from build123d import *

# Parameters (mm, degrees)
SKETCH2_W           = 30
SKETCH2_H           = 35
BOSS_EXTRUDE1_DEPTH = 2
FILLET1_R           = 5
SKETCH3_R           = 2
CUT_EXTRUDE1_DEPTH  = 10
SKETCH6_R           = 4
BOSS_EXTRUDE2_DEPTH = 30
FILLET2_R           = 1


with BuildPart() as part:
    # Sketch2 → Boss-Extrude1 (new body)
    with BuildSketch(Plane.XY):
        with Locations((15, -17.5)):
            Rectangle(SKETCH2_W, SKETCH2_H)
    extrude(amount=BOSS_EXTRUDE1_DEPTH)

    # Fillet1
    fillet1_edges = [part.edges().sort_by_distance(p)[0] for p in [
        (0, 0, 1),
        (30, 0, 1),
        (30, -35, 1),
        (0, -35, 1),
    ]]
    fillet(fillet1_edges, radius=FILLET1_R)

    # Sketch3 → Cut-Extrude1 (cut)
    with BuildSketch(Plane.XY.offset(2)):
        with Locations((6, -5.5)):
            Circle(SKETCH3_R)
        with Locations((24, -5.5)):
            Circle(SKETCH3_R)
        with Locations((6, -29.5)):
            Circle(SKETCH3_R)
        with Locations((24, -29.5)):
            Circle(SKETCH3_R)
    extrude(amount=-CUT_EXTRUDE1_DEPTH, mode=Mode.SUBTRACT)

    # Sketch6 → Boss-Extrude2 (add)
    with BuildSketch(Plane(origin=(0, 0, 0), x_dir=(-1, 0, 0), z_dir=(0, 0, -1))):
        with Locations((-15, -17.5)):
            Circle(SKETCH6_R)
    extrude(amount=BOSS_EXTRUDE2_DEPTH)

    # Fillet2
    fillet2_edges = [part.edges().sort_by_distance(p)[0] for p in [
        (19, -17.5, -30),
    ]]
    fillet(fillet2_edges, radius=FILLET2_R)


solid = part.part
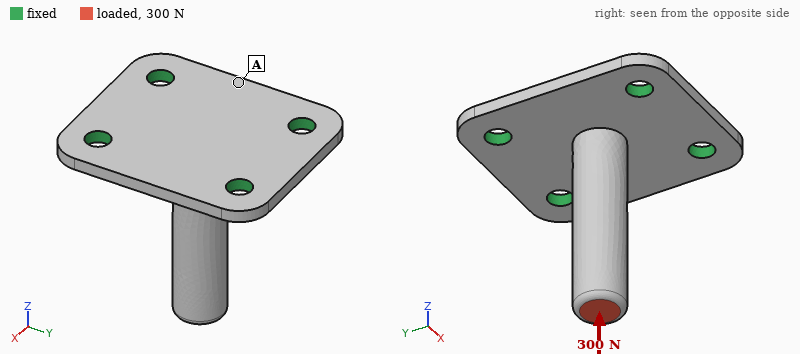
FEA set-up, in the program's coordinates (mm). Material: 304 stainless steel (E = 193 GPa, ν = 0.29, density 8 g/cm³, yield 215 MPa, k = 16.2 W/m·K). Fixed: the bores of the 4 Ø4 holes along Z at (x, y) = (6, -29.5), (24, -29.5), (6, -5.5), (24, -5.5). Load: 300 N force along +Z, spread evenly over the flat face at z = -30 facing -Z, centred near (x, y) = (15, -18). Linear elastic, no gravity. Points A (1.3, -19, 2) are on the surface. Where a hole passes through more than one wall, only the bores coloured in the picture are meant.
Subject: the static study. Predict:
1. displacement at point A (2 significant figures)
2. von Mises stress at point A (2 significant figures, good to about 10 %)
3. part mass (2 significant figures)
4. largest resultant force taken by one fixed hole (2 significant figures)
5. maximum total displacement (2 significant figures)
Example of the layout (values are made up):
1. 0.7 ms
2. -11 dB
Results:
1. 1.2 µm
2. 11 MPa
3. 28 g
4. 77 N
5. 6.9 µm
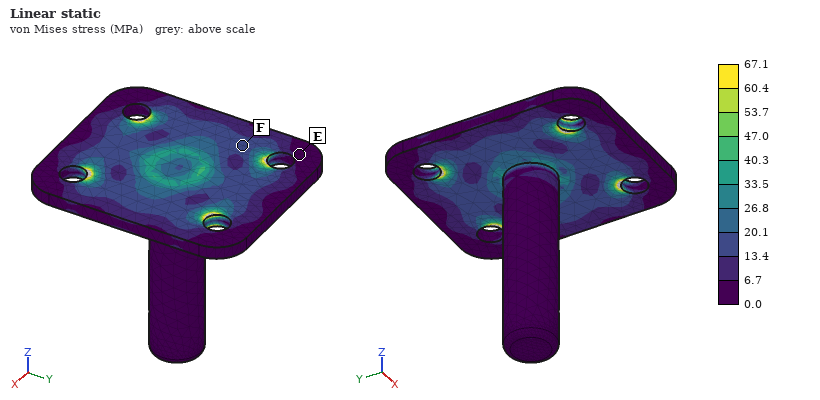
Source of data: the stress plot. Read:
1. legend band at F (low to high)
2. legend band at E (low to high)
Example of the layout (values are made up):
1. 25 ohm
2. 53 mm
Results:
1. 13.4 to 20.1 MPa
2. 0.0 to 6.7 MPa
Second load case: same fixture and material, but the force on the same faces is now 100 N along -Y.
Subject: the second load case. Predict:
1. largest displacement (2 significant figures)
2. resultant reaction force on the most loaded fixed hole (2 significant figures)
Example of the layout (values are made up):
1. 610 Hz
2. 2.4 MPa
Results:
1. 64 µm
2. 96 N
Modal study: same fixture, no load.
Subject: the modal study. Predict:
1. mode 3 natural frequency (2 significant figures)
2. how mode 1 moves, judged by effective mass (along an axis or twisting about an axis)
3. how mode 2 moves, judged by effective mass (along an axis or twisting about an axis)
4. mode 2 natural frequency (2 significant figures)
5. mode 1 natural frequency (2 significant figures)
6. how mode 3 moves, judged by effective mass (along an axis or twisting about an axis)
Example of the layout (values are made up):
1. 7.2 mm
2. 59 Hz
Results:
1. 9100 Hz
2. along X
3. along Y
4. 3300 Hz
5. 3100 Hz
6. along Z
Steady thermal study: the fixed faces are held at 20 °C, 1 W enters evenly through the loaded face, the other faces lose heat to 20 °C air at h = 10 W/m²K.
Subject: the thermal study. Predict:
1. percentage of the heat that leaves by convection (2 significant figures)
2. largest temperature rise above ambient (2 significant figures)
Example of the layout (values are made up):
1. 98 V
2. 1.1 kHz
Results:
1. 22 %
2. 41 K
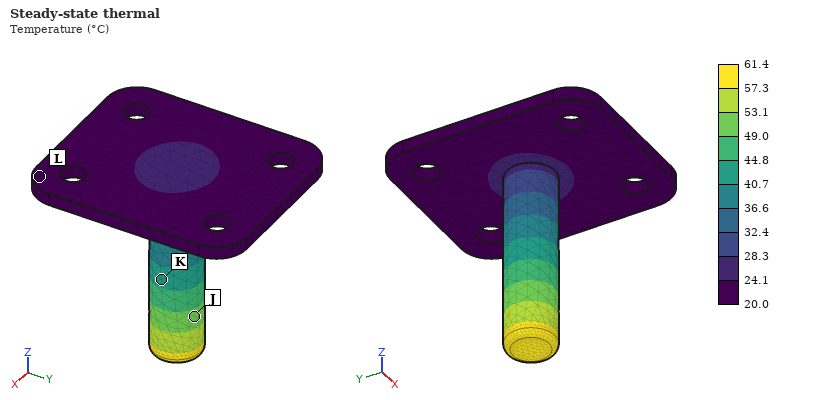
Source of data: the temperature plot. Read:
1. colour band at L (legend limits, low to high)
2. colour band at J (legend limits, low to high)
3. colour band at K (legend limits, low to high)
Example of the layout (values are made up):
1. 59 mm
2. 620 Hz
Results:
1. 20.0 to 24.1 °C
2. 49.0 to 53.1 °C
3. 40.7 to 44.8 °C
